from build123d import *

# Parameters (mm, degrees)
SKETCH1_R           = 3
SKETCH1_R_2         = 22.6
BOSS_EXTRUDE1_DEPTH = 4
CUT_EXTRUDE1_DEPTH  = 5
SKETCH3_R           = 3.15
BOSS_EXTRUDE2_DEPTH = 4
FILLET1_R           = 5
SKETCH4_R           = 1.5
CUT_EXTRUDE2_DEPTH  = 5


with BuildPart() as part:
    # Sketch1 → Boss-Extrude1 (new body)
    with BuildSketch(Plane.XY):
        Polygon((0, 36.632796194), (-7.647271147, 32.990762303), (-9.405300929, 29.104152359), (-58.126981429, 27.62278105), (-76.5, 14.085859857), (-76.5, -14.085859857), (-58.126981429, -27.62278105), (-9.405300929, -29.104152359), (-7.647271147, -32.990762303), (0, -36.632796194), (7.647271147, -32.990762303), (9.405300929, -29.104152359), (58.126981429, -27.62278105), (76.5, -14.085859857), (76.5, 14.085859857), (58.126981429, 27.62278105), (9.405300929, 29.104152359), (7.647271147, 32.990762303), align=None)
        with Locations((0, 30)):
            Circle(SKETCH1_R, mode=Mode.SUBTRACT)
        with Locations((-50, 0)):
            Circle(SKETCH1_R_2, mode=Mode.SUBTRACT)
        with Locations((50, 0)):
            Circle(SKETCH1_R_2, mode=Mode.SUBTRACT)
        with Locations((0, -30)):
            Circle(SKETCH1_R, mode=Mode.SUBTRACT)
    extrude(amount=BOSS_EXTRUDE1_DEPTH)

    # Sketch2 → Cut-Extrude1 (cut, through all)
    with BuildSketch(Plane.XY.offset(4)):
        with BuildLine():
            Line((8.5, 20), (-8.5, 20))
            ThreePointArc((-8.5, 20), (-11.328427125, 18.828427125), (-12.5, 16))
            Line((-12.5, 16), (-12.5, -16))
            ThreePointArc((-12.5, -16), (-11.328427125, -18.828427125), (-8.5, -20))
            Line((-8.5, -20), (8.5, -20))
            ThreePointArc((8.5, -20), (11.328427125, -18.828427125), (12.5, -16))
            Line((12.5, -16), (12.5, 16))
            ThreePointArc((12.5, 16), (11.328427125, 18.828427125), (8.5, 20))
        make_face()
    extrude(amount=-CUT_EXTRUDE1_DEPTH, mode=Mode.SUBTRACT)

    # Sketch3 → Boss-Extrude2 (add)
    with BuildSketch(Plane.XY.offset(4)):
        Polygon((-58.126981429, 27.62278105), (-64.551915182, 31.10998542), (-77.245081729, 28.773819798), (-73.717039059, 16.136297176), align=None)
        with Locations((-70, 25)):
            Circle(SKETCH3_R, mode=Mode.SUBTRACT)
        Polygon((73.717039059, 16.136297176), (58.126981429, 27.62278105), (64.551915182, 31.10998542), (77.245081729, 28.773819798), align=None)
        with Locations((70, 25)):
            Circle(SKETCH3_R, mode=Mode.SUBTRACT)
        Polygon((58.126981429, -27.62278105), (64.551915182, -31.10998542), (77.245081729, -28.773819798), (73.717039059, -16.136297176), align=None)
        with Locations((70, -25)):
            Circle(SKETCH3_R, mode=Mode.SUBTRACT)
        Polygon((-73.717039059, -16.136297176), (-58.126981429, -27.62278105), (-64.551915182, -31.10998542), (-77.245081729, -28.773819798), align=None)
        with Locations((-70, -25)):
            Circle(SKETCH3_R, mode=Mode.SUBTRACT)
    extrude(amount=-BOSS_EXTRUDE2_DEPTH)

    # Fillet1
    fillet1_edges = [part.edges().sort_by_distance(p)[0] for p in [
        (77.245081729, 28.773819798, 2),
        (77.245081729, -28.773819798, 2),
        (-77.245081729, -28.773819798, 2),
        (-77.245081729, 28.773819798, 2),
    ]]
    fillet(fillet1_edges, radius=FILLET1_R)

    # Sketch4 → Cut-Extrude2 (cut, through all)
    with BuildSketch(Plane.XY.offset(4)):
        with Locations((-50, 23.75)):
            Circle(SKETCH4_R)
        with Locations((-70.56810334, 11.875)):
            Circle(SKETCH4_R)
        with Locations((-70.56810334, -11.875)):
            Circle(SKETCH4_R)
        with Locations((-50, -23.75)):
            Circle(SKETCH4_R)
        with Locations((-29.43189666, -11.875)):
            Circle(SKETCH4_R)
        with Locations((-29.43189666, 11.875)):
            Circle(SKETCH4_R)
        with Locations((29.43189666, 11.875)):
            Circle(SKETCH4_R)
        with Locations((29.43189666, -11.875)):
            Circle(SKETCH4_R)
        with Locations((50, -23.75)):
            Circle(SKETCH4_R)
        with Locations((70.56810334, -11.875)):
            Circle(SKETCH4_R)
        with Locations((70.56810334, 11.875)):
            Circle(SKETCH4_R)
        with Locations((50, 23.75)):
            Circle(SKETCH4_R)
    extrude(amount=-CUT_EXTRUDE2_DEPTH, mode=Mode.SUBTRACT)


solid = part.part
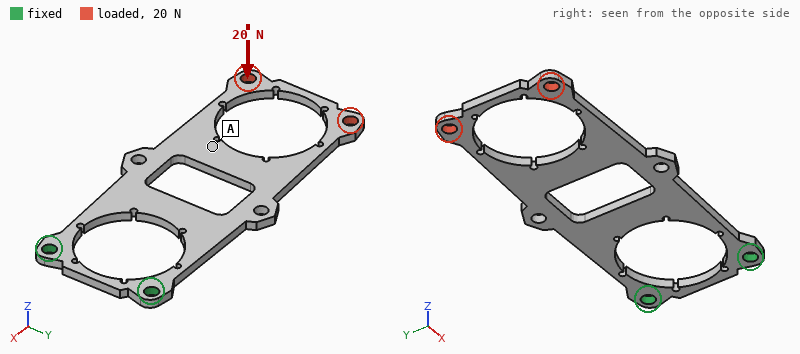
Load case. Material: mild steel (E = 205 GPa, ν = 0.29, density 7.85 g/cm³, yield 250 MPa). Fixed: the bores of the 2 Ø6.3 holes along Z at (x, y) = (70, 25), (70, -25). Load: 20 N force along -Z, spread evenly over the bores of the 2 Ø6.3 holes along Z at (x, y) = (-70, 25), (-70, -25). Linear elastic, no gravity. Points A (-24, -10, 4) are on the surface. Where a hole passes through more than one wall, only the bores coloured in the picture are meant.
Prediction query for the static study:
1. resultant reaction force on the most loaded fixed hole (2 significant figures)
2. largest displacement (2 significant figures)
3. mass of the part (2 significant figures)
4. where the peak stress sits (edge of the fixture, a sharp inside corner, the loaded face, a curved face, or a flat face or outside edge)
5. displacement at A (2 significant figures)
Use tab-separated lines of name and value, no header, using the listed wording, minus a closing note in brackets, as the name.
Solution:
resultant reaction force on the most loaded fixed hole	10 N
largest displacement	1.1 mm
mass of the part	140 g
where the peak stress sits	a curved face
displacement at A	0.59 mm
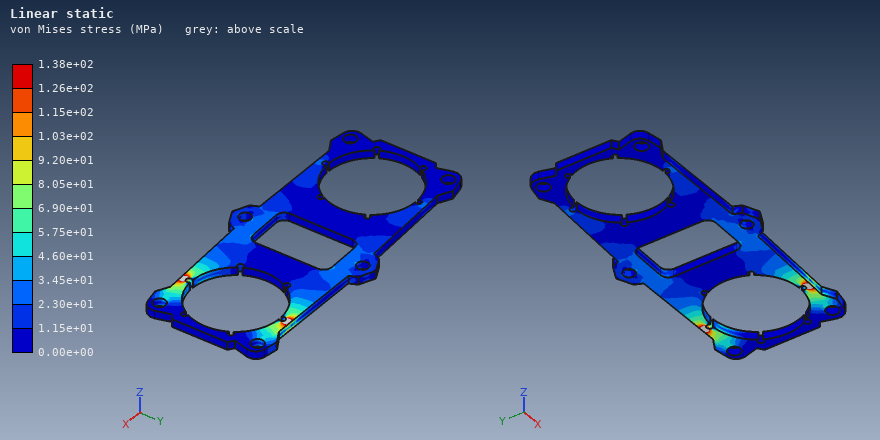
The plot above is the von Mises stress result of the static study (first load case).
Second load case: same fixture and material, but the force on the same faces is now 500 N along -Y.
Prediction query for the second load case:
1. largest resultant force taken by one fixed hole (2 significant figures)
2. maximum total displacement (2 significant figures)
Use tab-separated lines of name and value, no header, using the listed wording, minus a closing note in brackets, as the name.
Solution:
largest resultant force taken by one fixed hole	1.2 kN
maximum total displacement	0.22 mm
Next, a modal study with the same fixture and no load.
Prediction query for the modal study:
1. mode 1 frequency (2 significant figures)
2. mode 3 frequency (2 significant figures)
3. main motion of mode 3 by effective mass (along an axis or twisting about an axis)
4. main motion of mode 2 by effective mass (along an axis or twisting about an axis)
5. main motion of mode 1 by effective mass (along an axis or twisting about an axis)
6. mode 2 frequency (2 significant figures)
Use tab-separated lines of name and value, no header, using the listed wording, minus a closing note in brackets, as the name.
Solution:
mode 1 frequency	120 Hz
mode 3 frequency	730 Hz
main motion of mode 3 by effective mass	along Z
main motion of mode 2 by effective mass	twisting about X
main motion of mode 1 by effective mass	along Z
mode 2 frequency	610 Hz
